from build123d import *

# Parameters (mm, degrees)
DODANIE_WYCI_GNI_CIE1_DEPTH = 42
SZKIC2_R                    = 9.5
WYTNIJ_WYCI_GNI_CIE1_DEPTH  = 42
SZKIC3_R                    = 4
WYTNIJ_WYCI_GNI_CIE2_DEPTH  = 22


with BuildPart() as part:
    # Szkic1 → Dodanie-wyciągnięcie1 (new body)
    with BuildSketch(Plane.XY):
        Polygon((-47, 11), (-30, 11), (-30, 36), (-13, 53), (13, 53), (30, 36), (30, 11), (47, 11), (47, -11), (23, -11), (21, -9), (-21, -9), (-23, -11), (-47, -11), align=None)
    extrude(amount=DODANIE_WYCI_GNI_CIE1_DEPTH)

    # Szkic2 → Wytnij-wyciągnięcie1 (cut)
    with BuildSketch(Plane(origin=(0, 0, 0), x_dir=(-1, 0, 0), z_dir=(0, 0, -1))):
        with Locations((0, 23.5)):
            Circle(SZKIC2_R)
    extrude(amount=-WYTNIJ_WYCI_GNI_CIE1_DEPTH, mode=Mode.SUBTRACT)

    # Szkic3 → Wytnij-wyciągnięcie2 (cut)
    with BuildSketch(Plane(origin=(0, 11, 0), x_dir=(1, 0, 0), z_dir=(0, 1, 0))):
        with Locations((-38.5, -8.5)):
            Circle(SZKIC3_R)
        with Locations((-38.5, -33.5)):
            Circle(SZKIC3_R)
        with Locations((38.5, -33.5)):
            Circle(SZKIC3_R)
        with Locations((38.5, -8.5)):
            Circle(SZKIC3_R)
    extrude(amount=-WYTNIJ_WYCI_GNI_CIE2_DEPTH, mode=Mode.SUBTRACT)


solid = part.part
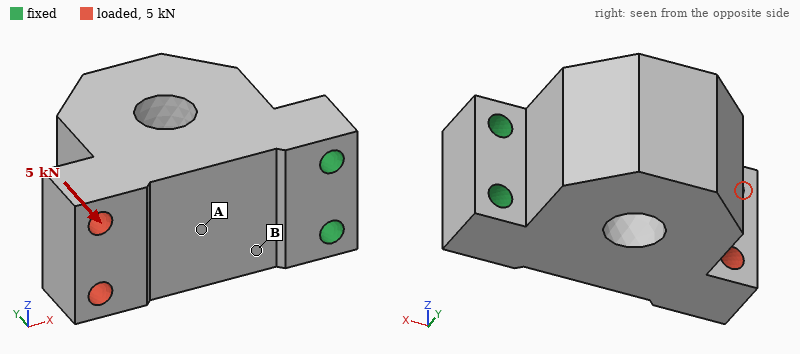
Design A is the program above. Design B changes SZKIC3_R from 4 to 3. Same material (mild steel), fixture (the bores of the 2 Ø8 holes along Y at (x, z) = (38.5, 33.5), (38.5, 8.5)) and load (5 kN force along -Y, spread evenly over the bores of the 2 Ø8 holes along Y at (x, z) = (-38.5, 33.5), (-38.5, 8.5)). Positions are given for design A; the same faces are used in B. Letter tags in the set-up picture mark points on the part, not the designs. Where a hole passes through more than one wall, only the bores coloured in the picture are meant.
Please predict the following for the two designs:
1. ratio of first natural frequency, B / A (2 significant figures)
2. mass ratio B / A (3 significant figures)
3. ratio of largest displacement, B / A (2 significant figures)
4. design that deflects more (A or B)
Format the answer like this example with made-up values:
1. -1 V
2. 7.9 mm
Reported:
1. 0.94
2. 1.01
3. 1.1
4. B
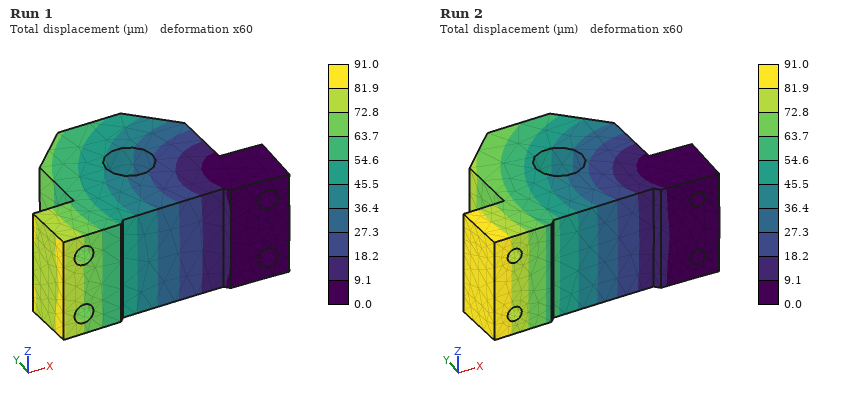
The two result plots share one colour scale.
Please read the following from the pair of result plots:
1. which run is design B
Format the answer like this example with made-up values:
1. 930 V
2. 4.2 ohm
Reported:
1. Run 2
